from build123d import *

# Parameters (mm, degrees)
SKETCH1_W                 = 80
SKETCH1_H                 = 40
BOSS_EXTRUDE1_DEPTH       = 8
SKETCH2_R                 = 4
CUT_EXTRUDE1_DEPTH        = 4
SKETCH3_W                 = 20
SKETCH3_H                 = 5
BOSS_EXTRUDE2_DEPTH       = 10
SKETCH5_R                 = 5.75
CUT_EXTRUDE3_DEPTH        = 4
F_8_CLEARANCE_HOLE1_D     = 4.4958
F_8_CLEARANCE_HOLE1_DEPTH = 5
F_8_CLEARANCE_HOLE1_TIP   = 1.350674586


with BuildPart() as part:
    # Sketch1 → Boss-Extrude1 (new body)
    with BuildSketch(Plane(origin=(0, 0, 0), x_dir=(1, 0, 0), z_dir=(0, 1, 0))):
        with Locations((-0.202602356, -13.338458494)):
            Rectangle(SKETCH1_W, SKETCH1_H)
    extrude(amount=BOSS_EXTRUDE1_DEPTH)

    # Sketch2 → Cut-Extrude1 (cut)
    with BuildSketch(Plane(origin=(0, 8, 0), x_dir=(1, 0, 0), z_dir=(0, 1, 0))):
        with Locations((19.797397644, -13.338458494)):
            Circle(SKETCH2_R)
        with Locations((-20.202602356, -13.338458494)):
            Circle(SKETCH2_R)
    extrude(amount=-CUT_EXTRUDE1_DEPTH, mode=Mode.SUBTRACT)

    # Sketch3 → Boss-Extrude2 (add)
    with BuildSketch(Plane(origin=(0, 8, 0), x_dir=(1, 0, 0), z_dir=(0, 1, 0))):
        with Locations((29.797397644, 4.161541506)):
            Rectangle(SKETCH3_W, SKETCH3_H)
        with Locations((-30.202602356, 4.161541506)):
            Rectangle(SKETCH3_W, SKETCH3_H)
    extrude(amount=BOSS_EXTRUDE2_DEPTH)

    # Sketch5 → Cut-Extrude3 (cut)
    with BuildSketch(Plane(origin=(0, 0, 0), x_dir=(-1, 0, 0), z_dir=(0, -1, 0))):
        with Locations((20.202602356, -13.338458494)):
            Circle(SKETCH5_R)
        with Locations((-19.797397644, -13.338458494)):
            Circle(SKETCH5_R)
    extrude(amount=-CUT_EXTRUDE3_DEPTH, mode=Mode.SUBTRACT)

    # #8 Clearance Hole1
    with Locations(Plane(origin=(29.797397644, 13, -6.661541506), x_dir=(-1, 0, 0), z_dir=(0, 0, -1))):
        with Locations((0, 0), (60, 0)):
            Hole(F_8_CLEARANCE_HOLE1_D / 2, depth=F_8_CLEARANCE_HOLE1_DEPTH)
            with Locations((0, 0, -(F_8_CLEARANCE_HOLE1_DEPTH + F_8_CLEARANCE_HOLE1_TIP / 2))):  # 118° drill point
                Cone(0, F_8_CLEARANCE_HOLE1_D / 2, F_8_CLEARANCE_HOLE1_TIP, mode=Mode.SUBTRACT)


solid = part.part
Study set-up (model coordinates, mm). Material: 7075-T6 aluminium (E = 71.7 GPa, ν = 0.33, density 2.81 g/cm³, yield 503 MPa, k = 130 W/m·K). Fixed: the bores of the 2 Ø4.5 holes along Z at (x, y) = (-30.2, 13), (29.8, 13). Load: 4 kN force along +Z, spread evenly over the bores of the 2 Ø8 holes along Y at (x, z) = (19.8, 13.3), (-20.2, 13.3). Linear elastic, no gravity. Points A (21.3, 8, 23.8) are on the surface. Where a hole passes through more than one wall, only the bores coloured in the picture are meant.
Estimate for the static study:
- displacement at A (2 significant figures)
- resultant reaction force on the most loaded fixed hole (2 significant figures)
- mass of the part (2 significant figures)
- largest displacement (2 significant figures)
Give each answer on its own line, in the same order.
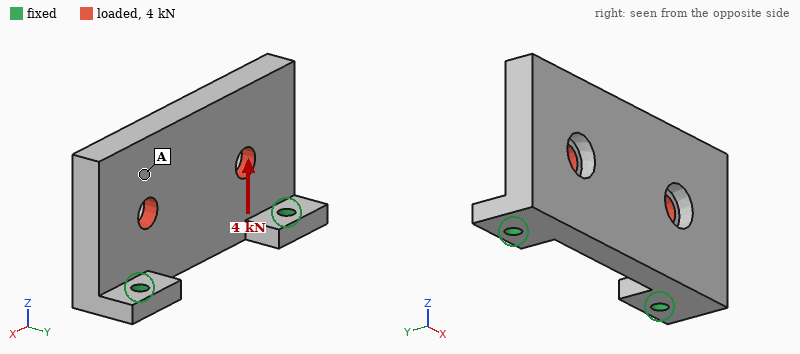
0.087 mm
2.0 kN
74 g
0.12 mm
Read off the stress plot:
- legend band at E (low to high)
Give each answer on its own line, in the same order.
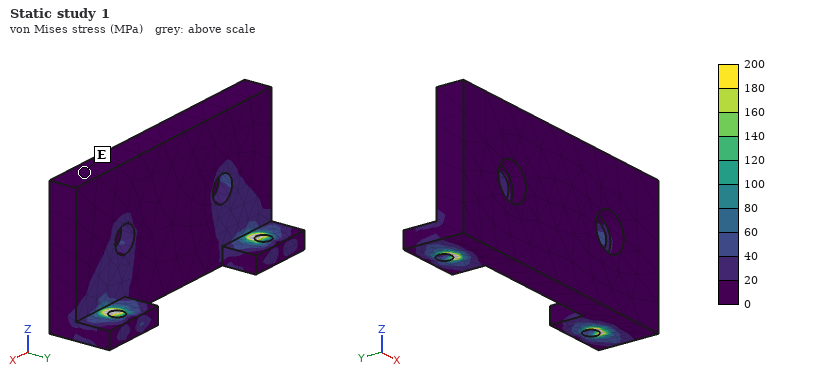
0 to 20 MPa
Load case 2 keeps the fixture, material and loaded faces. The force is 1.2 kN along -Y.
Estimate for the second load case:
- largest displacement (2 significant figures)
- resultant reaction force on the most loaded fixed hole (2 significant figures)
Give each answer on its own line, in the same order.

0.24 mm
660 N
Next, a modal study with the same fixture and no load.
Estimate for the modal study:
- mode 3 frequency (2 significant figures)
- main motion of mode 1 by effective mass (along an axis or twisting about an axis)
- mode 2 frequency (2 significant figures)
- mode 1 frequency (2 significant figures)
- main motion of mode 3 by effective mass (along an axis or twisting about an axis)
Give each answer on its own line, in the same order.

7600 Hz
along Y
4300 Hz
1600 Hz
along X
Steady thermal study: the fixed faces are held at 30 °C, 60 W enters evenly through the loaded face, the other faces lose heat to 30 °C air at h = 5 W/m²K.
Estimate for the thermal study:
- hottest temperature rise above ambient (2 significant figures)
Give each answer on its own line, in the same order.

44 K
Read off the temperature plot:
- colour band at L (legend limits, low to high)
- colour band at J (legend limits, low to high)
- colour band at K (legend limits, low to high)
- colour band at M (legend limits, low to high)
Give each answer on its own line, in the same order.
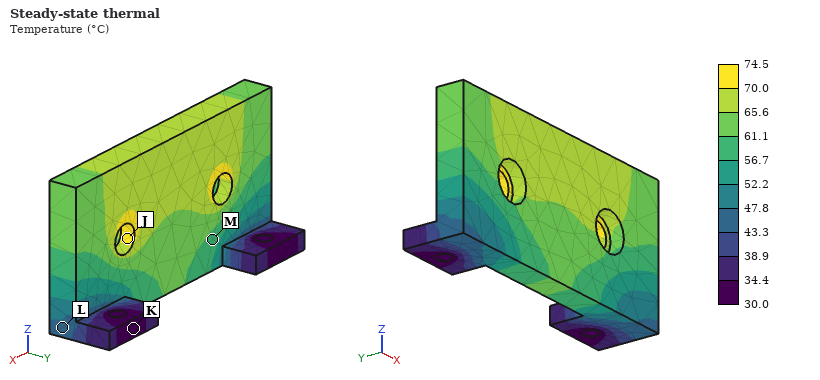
43.3 to 47.8 °C
70.0 to 74.5 °C
30.0 to 34.4 °C
56.7 to 61.1 °C
